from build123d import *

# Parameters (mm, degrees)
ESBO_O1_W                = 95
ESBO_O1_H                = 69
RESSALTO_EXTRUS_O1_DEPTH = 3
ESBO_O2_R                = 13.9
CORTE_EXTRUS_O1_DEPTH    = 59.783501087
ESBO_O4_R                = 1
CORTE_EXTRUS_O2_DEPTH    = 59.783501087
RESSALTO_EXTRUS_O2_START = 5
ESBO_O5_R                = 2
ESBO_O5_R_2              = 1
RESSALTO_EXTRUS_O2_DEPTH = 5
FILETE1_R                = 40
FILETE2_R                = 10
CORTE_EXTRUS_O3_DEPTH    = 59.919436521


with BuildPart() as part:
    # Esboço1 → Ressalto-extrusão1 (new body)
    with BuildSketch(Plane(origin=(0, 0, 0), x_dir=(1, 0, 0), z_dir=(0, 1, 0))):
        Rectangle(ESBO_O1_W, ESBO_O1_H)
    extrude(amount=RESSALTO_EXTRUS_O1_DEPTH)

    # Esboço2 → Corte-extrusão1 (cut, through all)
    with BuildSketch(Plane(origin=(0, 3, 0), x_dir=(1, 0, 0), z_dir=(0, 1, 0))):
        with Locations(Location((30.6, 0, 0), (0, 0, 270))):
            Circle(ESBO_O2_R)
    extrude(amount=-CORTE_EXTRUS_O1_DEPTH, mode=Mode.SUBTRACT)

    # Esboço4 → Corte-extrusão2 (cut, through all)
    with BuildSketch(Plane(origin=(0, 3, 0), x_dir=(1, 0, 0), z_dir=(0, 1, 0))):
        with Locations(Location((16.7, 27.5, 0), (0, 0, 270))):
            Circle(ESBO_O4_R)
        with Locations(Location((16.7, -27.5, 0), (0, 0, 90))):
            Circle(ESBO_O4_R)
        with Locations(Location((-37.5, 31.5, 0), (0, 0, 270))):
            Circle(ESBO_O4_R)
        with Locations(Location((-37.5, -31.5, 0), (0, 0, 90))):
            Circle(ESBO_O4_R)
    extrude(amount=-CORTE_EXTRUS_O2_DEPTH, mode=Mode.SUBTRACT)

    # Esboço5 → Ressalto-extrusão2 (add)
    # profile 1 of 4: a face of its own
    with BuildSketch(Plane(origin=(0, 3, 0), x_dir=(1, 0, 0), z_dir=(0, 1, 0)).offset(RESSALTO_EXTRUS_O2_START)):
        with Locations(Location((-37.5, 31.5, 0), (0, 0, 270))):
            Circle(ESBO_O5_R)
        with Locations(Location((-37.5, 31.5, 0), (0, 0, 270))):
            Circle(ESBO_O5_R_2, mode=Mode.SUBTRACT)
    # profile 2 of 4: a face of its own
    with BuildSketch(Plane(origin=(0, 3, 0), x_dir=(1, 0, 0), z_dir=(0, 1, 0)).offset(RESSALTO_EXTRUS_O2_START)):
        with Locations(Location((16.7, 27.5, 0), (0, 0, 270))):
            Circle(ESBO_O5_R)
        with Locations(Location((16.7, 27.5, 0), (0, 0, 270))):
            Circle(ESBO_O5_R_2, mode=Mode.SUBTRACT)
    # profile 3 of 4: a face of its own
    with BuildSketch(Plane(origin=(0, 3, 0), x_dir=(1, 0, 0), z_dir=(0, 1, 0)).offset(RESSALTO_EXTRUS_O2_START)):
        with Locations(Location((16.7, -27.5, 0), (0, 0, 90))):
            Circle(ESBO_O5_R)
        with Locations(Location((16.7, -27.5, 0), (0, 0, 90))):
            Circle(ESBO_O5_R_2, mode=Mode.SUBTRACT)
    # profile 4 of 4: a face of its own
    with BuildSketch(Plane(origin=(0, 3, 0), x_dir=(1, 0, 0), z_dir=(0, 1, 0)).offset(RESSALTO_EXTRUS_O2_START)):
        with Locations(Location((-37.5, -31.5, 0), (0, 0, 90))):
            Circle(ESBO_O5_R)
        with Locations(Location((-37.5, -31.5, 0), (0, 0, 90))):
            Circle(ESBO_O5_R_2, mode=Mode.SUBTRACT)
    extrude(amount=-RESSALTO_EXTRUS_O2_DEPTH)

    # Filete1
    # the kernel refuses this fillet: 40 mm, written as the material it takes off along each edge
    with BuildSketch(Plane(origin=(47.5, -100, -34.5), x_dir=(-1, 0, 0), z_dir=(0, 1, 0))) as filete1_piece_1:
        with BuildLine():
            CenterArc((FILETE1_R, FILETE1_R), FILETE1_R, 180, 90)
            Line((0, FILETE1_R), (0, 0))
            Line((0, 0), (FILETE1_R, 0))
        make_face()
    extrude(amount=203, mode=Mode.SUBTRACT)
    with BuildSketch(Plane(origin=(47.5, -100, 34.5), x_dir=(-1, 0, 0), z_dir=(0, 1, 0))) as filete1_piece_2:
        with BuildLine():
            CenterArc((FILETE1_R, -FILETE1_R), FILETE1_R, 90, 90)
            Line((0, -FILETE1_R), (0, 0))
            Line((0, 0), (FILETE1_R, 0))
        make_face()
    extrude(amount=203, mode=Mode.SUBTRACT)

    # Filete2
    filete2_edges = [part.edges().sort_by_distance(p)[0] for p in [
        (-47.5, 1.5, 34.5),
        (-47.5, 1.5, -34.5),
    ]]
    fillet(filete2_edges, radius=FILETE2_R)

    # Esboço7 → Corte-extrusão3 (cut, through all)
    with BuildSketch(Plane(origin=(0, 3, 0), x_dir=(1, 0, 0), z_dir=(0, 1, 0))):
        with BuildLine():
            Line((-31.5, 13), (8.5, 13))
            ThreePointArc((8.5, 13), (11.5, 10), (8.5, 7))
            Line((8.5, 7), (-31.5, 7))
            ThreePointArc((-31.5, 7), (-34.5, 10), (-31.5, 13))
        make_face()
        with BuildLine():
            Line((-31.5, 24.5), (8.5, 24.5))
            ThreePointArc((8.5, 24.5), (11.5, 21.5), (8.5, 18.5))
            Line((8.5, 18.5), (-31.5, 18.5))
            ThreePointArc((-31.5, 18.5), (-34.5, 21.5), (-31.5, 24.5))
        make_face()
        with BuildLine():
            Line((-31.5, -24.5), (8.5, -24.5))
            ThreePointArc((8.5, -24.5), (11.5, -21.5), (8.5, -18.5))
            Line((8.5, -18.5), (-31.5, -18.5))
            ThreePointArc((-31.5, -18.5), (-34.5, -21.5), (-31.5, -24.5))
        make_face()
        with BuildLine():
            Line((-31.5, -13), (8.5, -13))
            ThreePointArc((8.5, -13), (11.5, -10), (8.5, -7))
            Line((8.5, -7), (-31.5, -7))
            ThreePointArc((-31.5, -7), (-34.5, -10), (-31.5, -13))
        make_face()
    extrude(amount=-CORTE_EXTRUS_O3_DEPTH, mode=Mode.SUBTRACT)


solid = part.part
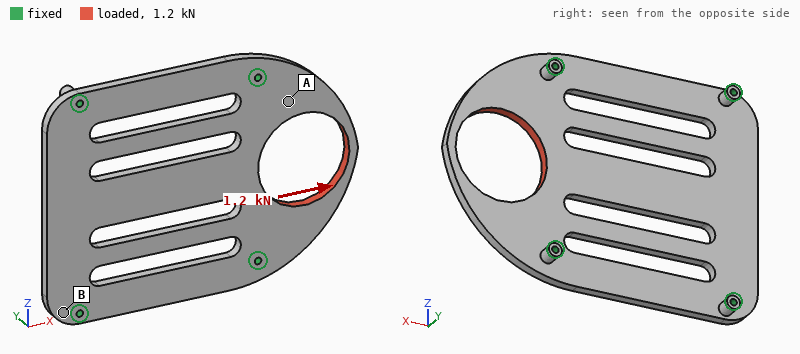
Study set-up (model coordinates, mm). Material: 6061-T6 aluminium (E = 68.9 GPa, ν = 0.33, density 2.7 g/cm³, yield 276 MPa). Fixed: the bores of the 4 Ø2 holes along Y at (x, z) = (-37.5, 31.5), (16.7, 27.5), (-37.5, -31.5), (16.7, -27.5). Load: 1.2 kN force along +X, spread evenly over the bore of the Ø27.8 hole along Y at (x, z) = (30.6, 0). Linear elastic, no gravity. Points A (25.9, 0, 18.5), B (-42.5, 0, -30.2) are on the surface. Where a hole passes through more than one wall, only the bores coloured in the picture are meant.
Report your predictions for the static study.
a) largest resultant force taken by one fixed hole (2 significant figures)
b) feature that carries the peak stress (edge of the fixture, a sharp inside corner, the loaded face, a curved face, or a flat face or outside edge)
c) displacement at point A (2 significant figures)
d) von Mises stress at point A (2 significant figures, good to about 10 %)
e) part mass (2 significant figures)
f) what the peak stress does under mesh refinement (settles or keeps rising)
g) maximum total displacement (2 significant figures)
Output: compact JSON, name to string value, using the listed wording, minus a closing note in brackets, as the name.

{"largest resultant force taken by one fixed hole": "520 N", "feature that carries the peak stress": "edge of the fixture", "displacement at point A": "7.4 µm", "von Mises stress at point A": "12 MPa", "part mass": "34 g", "what the peak stress does under mesh refinement": "keeps rising", "maximum total displacement": "13 µm"}
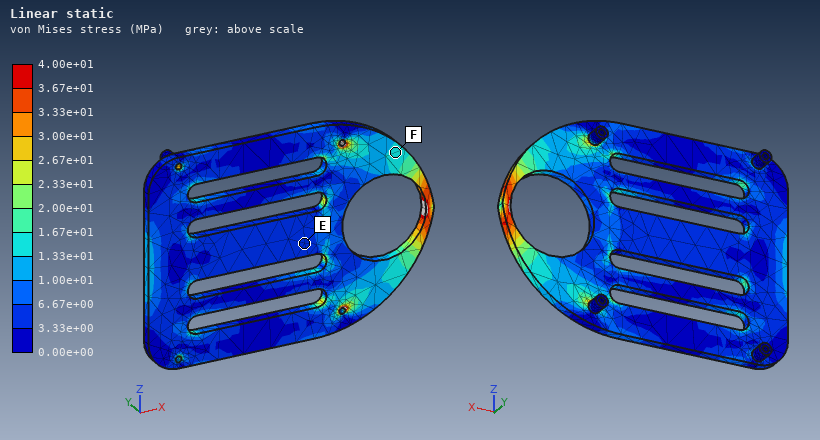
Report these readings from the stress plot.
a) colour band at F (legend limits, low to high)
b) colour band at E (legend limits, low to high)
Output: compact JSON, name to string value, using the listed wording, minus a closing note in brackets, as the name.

{"colour band at F": "1.33e+01 to 1.67e+01 MPa", "colour band at E": "3.33e+00 to 6.67e+00 MPa"}
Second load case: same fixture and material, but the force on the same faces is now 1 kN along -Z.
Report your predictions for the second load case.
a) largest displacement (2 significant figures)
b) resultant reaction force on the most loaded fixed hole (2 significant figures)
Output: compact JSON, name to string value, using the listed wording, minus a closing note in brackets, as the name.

{"largest displacement": "35 µm", "resultant reaction force on the most loaded fixed hole": "550 N"}
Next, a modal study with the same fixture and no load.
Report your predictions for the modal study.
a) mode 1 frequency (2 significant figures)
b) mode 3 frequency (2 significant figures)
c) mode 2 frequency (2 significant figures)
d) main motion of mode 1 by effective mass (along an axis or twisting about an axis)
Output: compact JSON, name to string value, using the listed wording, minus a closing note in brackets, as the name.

{"mode 1 frequency": "2500 Hz", "mode 3 frequency": "4000 Hz", "mode 2 frequency": "3100 Hz", "main motion of mode 1 by effective mass": "along Y"}
